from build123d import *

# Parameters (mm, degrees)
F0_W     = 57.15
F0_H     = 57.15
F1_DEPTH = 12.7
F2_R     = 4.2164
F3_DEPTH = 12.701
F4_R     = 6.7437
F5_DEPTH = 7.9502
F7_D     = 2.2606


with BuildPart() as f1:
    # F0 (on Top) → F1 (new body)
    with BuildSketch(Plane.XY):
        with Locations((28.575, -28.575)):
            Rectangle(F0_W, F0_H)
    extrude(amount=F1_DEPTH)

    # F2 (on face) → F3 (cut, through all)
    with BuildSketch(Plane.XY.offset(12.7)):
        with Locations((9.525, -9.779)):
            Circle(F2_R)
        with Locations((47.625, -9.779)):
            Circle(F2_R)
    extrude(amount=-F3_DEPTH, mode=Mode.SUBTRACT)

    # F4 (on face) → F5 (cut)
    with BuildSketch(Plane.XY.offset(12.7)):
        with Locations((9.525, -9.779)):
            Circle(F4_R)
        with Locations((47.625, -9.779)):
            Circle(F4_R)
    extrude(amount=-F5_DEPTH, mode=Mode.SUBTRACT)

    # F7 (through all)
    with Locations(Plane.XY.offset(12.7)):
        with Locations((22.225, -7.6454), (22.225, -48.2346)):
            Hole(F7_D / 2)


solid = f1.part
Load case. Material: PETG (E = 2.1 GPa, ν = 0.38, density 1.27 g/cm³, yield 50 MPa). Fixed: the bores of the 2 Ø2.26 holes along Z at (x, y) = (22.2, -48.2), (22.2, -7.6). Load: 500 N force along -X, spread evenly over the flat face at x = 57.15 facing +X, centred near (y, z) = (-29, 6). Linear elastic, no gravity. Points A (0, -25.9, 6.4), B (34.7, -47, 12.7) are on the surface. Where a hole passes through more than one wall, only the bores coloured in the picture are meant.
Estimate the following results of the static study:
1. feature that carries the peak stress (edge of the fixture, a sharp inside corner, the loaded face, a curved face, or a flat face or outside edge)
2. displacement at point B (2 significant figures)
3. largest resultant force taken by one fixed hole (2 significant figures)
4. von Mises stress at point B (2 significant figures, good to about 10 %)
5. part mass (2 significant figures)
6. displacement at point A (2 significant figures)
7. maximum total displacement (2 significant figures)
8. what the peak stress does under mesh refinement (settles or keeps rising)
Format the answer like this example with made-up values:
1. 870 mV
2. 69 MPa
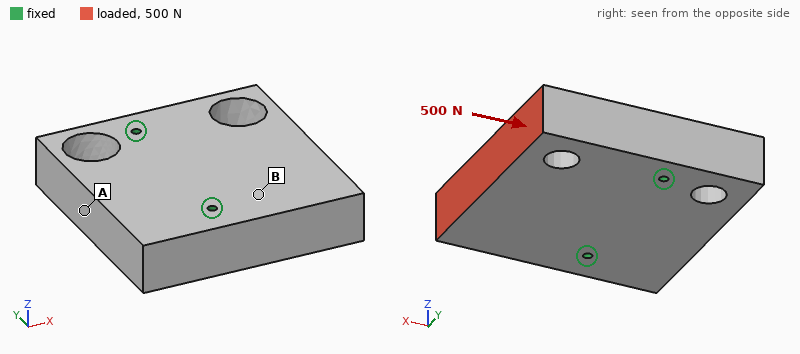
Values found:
1. edge of the fixture
2. 8.8 µm
3. 260 N
4. 0.97 MPa
5. 49 g
6. 7.8 µm
7. 43 µm
8. keeps rising
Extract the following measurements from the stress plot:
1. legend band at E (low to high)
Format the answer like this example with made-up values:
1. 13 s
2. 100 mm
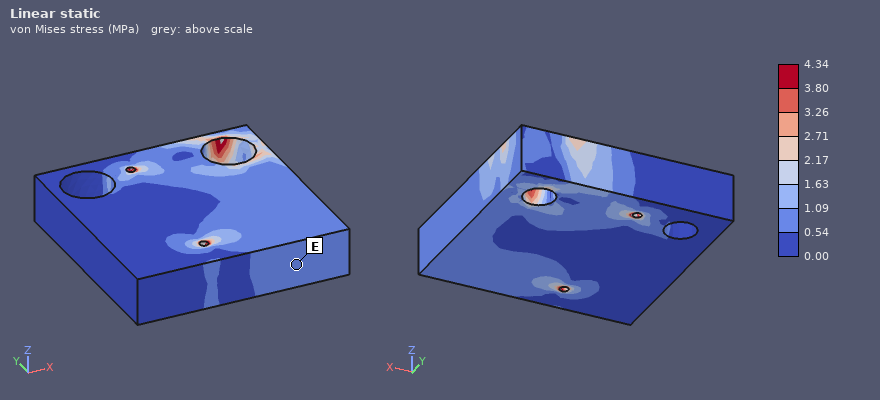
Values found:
1. 0.54 to 1.09 MPa
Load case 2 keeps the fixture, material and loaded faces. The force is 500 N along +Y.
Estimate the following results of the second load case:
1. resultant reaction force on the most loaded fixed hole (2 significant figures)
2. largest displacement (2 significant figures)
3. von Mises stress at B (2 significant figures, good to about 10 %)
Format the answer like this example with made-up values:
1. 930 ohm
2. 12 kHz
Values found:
1. 490 N
2. 0.10 mm
3. 1.6 MPa
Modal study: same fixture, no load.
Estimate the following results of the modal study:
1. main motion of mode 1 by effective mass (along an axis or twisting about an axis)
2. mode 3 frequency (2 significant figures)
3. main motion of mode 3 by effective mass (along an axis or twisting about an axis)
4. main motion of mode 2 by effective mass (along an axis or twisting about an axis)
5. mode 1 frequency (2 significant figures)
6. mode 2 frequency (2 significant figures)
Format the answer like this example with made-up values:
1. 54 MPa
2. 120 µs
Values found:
1. along Z
2. 3000 Hz
3. along Z
4. twisting about X
5. 1400 Hz
6. 2900 Hz
